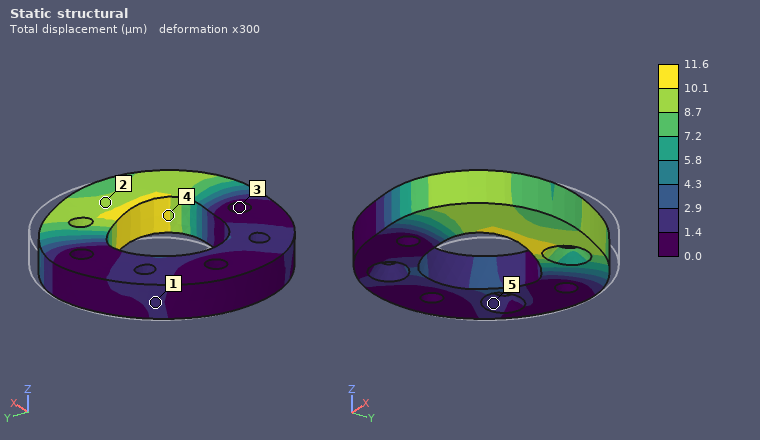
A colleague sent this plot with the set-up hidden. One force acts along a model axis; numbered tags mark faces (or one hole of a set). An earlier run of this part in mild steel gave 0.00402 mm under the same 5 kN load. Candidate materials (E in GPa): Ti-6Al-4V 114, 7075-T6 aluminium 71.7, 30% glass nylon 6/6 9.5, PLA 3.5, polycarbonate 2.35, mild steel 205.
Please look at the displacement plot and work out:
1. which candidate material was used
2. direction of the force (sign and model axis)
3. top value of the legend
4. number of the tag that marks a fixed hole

7075-T6 aluminium
-Y
11.6 µm
3
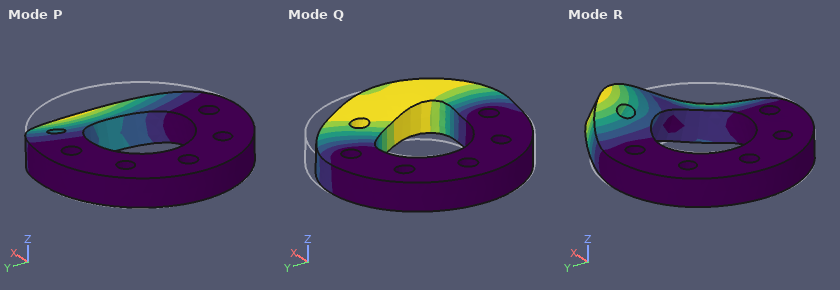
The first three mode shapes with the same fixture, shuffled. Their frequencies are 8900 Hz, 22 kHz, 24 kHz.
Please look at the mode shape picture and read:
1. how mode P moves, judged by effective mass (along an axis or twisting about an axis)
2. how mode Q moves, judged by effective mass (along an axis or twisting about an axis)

along Z
along Y
